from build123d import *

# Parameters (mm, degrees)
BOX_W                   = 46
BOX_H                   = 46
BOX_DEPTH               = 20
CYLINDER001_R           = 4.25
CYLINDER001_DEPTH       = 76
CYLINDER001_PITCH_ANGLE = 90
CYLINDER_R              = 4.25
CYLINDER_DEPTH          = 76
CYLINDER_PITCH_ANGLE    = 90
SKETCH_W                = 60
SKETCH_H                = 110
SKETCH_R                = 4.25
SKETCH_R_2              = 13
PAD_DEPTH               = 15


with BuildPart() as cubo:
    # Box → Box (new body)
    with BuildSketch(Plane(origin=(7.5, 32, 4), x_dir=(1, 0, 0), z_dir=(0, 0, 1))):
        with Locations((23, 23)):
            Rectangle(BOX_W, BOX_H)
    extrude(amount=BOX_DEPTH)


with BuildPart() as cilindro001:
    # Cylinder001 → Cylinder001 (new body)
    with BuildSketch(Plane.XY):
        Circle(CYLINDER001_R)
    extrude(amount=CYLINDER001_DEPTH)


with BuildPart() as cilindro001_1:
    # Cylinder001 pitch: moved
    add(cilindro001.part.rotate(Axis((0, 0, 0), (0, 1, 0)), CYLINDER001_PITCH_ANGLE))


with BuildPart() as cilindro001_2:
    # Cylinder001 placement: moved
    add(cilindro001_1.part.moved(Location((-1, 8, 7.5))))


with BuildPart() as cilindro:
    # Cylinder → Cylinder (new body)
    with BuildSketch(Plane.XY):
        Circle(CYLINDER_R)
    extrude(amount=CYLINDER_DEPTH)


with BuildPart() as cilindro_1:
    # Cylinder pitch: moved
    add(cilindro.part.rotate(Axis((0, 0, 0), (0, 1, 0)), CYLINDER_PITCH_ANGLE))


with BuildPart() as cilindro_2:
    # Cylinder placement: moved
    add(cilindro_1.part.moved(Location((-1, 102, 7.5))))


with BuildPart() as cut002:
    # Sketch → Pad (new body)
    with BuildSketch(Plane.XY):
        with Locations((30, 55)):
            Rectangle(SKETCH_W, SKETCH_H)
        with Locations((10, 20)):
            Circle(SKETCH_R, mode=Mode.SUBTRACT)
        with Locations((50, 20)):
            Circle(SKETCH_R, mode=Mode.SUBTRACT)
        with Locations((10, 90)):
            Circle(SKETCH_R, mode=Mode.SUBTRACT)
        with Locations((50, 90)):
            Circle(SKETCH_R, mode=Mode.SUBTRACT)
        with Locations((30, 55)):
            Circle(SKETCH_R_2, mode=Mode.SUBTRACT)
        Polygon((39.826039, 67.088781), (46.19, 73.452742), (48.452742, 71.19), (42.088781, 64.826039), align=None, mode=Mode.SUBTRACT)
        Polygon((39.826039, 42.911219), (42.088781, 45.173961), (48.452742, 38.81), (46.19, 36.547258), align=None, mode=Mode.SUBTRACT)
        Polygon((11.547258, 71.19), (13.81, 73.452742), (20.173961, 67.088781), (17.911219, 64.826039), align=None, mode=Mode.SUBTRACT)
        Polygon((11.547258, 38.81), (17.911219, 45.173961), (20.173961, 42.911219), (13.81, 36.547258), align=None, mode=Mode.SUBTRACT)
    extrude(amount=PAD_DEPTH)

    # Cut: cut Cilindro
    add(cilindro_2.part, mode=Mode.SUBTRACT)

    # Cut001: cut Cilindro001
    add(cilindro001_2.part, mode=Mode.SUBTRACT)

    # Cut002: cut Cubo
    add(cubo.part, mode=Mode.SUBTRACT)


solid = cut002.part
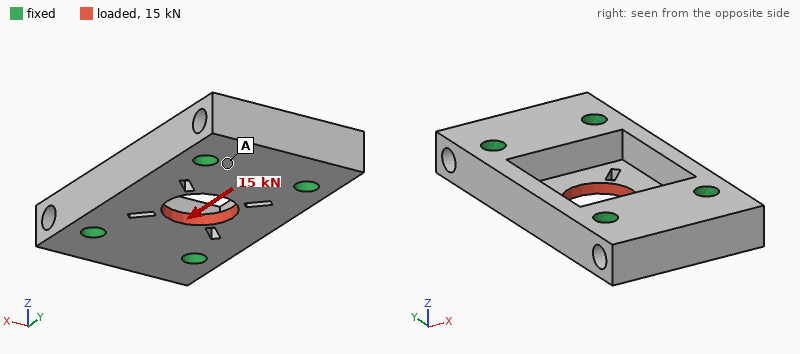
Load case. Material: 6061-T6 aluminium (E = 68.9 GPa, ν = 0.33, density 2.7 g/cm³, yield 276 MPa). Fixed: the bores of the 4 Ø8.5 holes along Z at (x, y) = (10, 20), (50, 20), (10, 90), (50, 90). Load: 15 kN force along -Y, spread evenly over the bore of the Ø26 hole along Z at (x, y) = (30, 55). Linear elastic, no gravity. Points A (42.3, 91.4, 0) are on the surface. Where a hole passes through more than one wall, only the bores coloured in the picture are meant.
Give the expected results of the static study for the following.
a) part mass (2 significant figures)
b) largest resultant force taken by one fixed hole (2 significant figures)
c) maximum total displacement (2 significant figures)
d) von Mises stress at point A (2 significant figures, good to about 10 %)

170 g
3.9 kN
23 µm
17 MPa
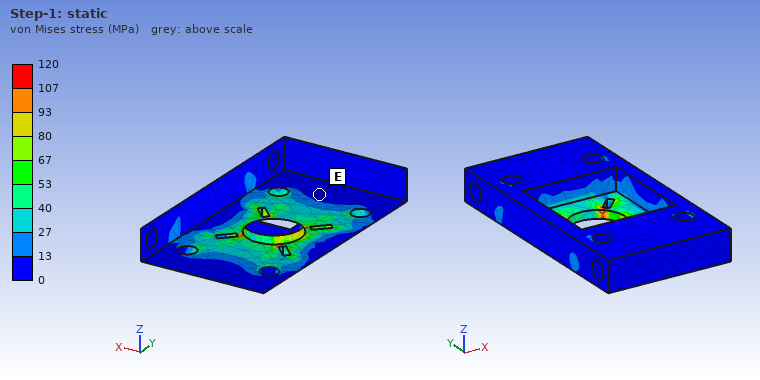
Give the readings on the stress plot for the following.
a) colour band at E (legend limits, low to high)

0 to 13 MPa
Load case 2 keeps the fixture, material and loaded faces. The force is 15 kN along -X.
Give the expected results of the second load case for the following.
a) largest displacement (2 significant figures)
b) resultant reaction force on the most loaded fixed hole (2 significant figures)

44 µm
4.5 kN
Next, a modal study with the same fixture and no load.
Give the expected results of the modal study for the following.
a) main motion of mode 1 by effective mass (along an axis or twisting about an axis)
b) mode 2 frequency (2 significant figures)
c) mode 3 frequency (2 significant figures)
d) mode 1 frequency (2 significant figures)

along Z
14 kHz
15 kHz
13 kHz
